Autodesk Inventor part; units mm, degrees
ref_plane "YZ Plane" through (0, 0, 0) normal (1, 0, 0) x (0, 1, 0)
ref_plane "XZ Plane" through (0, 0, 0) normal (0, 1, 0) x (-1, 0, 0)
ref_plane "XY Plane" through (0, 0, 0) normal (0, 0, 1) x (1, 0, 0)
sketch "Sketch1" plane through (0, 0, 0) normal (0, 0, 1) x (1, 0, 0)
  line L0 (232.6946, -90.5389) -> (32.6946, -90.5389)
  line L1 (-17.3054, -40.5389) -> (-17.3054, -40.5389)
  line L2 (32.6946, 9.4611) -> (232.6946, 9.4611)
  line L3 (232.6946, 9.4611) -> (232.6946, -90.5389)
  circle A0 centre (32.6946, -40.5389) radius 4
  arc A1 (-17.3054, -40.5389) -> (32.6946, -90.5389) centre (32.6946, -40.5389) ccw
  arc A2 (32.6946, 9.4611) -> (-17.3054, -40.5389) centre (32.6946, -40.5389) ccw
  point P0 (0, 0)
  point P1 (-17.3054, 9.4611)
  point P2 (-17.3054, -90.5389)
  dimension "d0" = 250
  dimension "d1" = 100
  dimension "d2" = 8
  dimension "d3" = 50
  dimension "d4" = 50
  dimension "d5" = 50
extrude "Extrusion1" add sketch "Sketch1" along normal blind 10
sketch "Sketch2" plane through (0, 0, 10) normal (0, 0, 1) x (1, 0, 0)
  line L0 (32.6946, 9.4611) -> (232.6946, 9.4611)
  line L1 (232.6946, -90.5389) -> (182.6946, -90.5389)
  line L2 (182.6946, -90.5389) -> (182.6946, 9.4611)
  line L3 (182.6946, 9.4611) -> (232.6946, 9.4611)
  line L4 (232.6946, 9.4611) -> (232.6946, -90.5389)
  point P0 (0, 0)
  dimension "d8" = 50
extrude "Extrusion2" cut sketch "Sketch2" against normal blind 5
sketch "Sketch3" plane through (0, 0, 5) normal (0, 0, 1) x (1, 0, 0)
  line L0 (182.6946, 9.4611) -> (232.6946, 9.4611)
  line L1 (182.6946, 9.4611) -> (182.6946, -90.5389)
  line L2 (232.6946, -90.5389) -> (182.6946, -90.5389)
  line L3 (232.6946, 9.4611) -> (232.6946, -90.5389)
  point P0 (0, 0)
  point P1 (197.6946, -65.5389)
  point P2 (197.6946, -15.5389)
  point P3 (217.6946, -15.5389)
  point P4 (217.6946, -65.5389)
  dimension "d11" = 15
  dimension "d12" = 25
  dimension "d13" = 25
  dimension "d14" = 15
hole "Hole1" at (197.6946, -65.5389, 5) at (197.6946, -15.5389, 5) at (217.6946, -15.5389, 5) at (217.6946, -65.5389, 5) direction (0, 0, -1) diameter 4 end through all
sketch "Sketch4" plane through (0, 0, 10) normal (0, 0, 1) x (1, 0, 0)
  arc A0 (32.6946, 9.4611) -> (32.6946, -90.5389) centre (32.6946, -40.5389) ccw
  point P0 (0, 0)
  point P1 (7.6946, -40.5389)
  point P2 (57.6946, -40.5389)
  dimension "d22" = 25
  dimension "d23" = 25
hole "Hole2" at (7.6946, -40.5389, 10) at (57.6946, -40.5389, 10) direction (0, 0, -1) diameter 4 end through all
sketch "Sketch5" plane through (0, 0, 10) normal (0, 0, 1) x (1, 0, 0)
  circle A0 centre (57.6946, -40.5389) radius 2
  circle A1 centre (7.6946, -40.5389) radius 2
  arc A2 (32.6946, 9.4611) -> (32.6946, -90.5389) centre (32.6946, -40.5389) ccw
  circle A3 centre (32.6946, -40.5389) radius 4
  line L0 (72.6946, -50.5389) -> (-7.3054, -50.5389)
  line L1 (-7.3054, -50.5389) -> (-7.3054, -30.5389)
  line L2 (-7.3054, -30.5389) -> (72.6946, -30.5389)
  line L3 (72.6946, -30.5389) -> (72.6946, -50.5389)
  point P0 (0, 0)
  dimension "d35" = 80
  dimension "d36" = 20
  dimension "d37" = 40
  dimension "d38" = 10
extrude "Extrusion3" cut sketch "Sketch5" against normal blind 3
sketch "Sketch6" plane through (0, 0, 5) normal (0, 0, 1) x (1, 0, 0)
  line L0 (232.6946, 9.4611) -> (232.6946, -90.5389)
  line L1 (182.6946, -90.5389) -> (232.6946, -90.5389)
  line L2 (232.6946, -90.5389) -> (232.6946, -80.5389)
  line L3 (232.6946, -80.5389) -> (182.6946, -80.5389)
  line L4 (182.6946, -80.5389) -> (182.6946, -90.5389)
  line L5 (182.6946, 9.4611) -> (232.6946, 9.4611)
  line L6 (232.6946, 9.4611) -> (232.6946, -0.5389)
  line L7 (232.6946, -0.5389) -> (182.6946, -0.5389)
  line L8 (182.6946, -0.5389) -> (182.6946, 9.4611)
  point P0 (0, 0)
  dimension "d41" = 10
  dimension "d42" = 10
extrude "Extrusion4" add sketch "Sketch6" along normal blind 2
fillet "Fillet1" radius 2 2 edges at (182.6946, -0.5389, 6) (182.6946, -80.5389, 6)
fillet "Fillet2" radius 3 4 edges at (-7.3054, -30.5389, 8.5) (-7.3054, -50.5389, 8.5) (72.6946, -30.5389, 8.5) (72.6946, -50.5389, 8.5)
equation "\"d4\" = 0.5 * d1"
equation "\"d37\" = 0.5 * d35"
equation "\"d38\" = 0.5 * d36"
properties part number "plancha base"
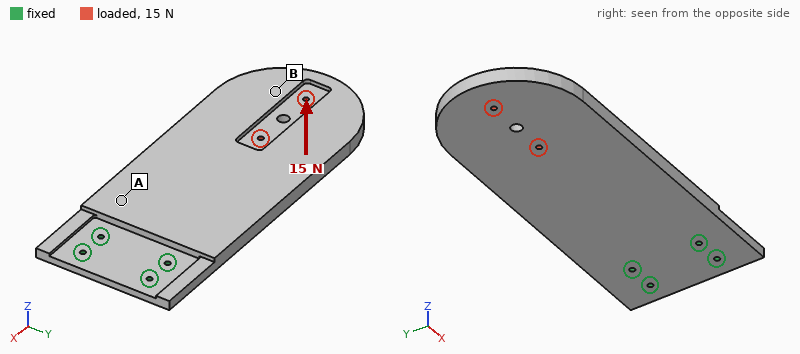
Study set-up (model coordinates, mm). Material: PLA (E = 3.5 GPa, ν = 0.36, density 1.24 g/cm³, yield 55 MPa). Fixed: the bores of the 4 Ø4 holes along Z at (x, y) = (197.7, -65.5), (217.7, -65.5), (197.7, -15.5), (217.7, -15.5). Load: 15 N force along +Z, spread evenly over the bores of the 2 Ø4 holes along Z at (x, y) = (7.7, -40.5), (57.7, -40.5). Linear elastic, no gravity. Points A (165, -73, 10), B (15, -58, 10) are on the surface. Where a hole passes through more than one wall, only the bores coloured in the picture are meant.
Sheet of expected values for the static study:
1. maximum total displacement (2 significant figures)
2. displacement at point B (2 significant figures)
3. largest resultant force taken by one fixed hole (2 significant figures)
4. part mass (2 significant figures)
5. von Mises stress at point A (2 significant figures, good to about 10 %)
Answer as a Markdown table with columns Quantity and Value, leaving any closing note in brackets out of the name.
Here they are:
| Quantity | Value |
|---|---|
| maximum total displacement | 2.8 mm |
| displacement at point B | 2.3 mm |
| largest resultant force taken by one fixed hole | 45 N |
| part mass | 260 g |
| von Mises stress at point A | 1.2 MPa |
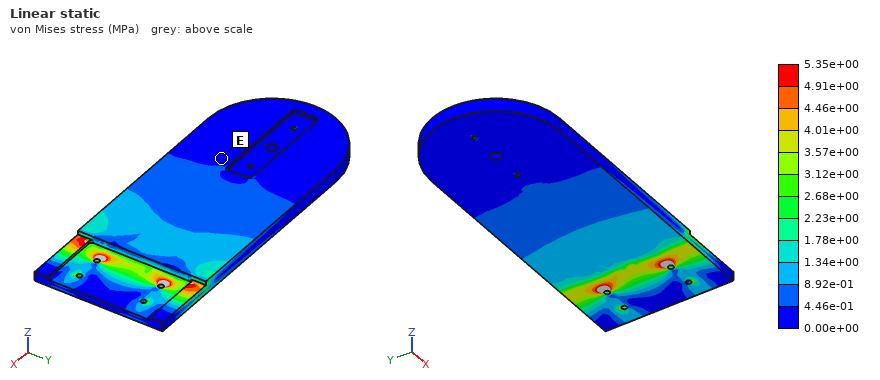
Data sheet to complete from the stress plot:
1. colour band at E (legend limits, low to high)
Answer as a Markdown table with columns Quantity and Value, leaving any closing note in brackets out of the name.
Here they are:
| Quantity | Value |
|---|---|
| colour band at E | 0.00e+00 to 4.46e-01 MPa |
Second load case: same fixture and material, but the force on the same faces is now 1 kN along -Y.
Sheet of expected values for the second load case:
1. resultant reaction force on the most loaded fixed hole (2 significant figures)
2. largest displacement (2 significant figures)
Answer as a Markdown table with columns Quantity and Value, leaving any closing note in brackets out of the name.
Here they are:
| Quantity | Value |
|---|---|
| resultant reaction force on the most loaded fixed hole | 2.1 kN |
| largest displacement | 1.9 mm |
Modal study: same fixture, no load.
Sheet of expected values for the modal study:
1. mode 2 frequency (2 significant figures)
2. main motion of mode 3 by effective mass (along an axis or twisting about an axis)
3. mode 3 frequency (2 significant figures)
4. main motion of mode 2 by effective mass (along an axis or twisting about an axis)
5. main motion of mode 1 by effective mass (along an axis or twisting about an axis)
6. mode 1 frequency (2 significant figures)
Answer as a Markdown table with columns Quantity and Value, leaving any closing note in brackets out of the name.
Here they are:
| Quantity | Value |
|---|---|
| mode 2 frequency | 240 Hz |
| main motion of mode 3 by effective mass | along Z |
| mode 3 frequency | 320 Hz |
| main motion of mode 2 by effective mass | twisting about X |
| main motion of mode 1 by effective mass | along Z |
| mode 1 frequency | 40 Hz |
